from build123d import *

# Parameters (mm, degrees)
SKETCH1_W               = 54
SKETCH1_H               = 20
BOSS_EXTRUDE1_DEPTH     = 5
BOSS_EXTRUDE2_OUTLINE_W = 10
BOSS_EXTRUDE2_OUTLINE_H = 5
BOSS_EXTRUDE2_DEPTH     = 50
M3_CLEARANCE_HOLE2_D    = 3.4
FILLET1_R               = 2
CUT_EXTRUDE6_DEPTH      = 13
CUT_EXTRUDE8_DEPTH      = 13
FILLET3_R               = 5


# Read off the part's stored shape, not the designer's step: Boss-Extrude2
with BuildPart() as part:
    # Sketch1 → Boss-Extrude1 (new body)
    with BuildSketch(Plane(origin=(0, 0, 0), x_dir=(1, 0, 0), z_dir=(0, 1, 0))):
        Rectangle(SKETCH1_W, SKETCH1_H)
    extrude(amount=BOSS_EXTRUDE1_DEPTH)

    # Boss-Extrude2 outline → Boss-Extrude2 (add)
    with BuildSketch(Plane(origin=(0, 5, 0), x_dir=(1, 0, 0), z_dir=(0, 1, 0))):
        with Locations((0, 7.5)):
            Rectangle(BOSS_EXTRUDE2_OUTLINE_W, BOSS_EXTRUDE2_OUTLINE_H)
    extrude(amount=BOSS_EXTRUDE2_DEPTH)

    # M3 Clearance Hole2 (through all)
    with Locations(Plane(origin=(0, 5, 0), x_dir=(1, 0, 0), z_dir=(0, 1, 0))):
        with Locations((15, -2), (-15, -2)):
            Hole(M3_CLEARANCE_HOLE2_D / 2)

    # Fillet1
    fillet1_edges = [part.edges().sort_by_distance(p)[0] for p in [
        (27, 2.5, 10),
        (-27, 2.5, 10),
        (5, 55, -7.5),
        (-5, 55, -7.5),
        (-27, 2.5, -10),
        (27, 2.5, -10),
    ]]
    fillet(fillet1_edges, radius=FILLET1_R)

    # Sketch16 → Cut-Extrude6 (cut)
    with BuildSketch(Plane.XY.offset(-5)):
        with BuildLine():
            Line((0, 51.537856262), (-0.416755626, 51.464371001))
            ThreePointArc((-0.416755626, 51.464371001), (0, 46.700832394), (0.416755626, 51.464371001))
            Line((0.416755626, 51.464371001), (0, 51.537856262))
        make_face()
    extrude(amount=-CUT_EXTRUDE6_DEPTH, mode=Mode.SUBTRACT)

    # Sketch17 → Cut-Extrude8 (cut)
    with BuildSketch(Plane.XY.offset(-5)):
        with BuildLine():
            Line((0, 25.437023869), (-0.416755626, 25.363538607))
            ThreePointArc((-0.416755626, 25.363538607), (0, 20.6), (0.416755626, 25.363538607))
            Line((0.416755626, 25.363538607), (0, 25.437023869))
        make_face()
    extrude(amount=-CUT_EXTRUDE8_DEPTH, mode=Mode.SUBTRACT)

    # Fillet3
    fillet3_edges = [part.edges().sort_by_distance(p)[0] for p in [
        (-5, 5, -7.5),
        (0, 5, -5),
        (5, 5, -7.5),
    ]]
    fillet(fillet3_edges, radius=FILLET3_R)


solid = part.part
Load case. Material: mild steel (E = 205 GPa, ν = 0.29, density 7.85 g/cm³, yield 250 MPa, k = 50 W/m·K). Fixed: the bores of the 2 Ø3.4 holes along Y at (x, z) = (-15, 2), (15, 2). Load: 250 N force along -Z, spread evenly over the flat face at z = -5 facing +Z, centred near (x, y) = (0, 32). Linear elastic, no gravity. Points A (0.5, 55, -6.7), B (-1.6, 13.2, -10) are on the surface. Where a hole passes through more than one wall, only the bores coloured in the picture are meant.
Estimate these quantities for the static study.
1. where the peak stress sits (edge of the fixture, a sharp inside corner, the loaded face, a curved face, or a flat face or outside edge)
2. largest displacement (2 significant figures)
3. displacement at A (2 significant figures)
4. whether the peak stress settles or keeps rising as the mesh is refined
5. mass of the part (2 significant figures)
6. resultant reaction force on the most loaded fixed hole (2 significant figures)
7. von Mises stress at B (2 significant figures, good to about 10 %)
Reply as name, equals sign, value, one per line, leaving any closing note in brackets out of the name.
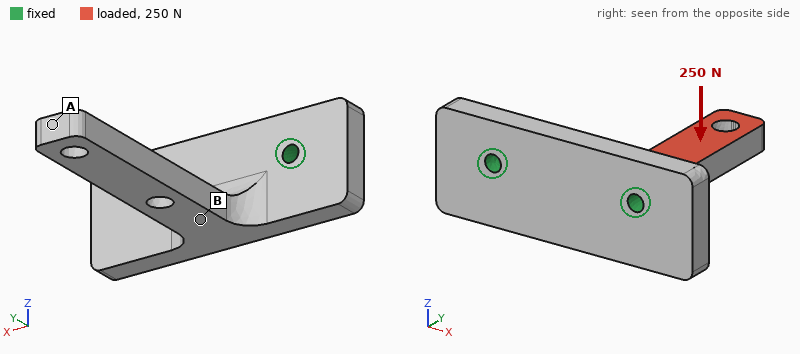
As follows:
where the peak stress sits = a sharp inside corner
largest displacement = 0.26 mm
displacement at A = 0.26 mm
whether the peak stress settles or keeps rising as the mesh is refined = keeps rising
mass of the part = 61 g
resultant reaction force on the most loaded fixed hole = 130 N
von Mises stress at B = 110 MPa
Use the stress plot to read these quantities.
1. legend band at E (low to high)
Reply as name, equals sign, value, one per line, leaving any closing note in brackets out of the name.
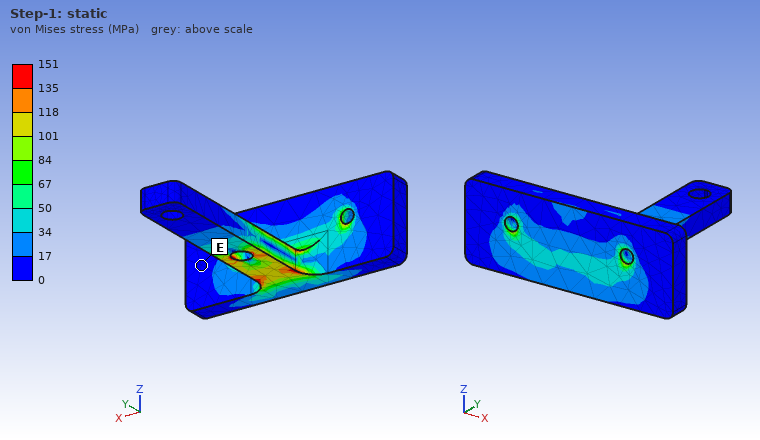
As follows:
legend band at E = 0 to 17 MPa
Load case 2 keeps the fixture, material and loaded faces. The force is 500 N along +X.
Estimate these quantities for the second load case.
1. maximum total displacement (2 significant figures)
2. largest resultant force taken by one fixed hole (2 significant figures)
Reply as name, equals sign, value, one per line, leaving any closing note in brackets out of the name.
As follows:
maximum total displacement = 0.14 mm
largest resultant force taken by one fixed hole = 650 N
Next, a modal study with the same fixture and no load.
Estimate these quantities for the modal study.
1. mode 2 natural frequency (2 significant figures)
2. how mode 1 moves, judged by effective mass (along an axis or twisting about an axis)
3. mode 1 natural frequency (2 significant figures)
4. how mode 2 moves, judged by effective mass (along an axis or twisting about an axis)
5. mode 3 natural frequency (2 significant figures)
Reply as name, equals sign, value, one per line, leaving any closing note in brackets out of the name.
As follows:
mode 2 natural frequency = 3000 Hz
how mode 1 moves, judged by effective mass = along Z
mode 1 natural frequency = 1500 Hz
how mode 2 moves, judged by effective mass = along X
mode 3 natural frequency = 8000 Hz
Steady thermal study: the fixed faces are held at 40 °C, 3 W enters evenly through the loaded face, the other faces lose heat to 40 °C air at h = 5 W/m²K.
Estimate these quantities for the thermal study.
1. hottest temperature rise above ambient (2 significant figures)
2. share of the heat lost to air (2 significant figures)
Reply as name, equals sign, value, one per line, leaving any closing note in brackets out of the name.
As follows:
hottest temperature rise above ambient = 39 K
share of the heat lost to air = 6.3 %
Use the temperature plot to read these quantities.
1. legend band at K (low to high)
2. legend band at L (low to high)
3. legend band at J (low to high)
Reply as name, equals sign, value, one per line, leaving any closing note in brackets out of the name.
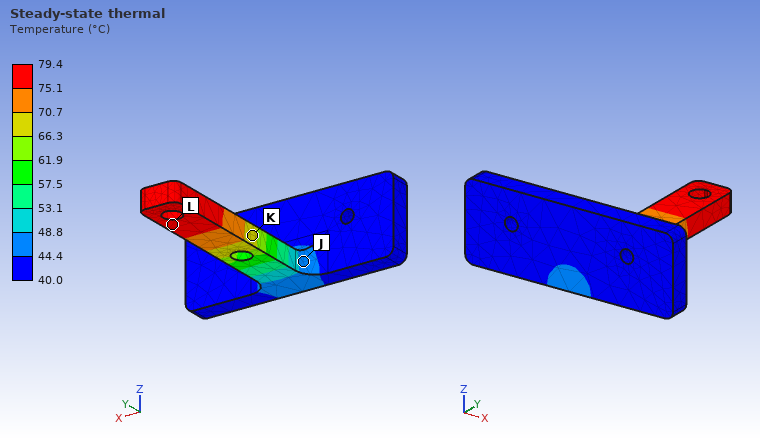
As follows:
legend band at K = 66.3 to 70.7 °C
legend band at L = 75.1 to 79.4 °C
legend band at J = 44.4 to 48.8 °C
